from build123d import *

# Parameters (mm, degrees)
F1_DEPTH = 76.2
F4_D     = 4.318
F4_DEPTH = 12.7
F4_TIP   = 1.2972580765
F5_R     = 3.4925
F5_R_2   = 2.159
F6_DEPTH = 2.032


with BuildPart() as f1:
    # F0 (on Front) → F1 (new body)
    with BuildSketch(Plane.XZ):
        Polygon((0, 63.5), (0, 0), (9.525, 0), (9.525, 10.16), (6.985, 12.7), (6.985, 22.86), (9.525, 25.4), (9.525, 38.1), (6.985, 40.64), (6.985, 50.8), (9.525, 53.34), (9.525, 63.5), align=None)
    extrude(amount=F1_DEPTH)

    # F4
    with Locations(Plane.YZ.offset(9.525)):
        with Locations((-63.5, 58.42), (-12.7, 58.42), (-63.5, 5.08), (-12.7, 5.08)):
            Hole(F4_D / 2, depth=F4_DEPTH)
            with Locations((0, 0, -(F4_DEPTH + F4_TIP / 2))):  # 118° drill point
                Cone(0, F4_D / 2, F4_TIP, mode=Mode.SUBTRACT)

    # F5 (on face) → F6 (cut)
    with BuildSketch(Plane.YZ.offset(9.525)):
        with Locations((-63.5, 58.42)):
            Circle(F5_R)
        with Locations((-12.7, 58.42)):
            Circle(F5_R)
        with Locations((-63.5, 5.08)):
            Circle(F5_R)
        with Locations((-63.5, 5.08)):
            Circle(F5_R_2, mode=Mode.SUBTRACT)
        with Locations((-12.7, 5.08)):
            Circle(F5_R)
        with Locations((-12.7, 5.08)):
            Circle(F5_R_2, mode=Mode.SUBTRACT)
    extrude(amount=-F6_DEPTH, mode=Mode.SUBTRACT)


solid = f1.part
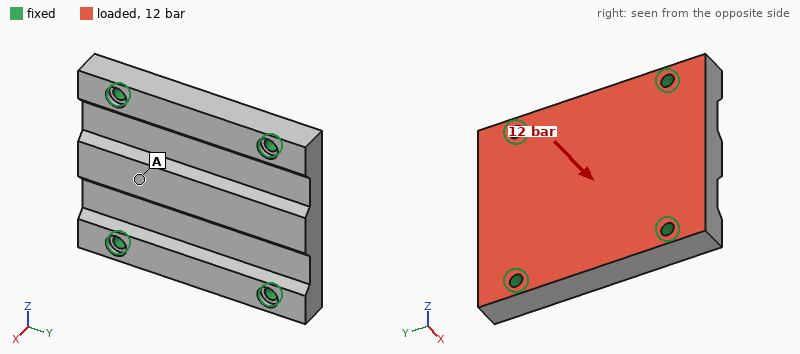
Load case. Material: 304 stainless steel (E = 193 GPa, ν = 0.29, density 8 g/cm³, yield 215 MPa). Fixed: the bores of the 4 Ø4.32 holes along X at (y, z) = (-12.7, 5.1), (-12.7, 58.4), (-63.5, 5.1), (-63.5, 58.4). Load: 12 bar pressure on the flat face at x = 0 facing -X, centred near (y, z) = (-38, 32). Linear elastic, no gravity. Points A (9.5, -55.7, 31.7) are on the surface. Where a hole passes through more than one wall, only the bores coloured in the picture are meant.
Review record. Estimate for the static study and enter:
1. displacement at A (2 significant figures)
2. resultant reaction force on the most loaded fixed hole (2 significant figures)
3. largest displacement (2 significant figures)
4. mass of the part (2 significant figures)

6.7 µm
1.4 kN
8.1 µm
320 g
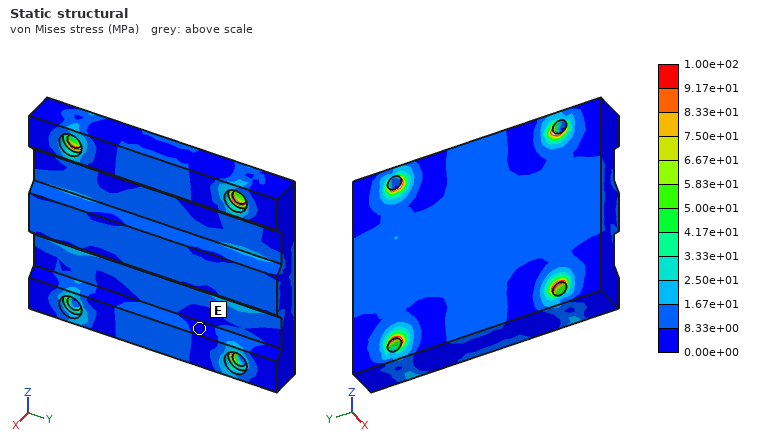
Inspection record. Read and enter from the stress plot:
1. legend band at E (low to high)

0.00e+00 to 8.33e+00 MPa
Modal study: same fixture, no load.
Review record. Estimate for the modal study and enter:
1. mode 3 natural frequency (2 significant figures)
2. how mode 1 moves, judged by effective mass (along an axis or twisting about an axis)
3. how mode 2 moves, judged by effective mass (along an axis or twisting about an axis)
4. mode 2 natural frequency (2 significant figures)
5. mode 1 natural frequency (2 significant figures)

13 kHz
along X
twisting about Z
12 kHz
8800 Hz
